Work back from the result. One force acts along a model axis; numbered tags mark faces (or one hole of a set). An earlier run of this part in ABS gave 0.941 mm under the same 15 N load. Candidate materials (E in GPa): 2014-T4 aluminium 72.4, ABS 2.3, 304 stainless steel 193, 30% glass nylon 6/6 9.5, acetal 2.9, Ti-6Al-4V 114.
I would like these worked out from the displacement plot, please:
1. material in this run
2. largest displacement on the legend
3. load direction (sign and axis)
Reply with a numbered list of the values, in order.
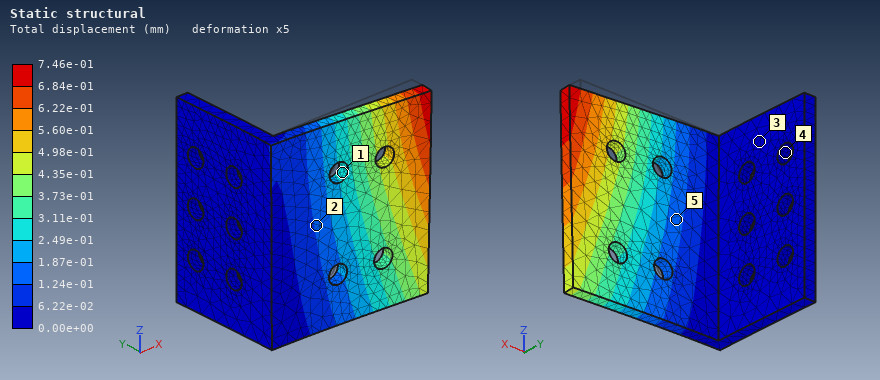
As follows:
1. acetal
2. 7.46e-01 mm
3. -Y
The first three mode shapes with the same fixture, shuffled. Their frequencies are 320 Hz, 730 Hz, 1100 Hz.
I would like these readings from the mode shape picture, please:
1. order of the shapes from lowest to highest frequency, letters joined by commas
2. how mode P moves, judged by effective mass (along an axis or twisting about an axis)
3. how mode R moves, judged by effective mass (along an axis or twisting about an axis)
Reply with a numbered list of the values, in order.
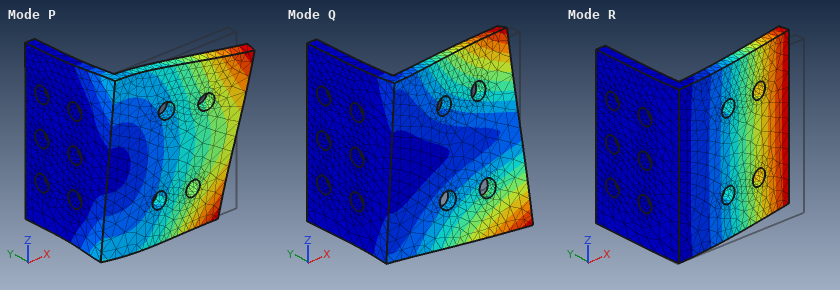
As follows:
1. R, Q, P
2. along Z
3. along Y
